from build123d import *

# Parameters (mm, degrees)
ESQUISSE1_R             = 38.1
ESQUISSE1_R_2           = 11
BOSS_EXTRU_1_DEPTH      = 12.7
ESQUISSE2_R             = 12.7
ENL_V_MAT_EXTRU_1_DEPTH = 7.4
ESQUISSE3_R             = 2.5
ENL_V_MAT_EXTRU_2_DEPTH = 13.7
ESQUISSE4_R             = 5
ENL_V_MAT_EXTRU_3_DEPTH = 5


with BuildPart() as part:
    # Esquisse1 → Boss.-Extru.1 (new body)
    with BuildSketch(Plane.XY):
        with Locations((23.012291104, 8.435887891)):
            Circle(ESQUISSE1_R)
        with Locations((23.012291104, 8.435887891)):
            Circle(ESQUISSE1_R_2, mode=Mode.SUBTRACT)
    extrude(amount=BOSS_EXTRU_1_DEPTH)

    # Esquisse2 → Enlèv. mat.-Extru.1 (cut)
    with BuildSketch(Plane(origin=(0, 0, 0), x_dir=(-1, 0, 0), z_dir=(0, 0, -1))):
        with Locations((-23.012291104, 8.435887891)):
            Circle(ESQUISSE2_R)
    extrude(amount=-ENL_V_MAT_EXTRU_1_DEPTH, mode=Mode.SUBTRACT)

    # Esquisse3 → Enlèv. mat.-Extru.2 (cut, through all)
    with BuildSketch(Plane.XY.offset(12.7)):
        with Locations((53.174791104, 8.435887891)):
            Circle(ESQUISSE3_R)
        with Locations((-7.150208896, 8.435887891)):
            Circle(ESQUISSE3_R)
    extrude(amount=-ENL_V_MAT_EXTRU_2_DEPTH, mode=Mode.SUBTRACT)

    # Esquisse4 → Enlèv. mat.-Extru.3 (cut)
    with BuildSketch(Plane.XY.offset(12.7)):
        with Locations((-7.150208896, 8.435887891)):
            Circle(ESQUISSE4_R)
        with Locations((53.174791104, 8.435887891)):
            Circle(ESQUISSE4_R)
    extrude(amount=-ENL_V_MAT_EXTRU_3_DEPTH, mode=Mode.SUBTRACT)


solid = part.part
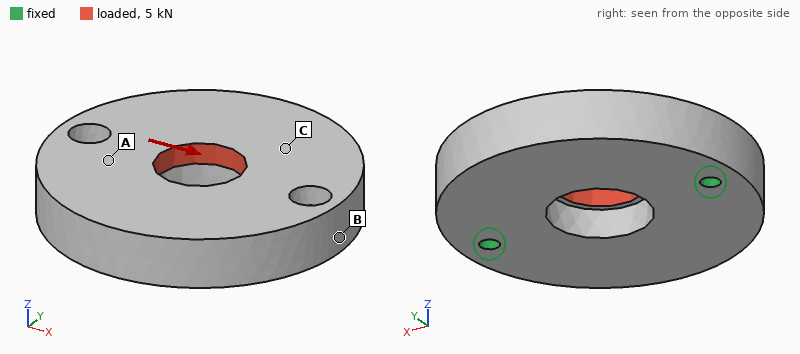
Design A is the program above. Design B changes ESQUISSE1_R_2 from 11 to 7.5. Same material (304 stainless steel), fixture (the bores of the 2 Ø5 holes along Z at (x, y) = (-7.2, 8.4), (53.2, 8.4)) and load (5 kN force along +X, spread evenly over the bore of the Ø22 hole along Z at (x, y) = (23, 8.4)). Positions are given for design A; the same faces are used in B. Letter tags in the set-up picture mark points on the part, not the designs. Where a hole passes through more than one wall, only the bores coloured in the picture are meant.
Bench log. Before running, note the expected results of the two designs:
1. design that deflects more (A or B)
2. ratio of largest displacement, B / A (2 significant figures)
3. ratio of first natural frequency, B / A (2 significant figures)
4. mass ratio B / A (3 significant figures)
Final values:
B
1.2
1.00
1.02
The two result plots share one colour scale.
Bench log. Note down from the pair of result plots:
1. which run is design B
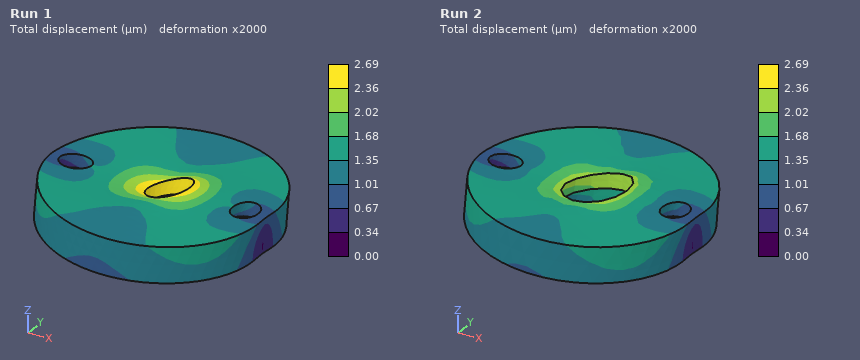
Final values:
Run 1
